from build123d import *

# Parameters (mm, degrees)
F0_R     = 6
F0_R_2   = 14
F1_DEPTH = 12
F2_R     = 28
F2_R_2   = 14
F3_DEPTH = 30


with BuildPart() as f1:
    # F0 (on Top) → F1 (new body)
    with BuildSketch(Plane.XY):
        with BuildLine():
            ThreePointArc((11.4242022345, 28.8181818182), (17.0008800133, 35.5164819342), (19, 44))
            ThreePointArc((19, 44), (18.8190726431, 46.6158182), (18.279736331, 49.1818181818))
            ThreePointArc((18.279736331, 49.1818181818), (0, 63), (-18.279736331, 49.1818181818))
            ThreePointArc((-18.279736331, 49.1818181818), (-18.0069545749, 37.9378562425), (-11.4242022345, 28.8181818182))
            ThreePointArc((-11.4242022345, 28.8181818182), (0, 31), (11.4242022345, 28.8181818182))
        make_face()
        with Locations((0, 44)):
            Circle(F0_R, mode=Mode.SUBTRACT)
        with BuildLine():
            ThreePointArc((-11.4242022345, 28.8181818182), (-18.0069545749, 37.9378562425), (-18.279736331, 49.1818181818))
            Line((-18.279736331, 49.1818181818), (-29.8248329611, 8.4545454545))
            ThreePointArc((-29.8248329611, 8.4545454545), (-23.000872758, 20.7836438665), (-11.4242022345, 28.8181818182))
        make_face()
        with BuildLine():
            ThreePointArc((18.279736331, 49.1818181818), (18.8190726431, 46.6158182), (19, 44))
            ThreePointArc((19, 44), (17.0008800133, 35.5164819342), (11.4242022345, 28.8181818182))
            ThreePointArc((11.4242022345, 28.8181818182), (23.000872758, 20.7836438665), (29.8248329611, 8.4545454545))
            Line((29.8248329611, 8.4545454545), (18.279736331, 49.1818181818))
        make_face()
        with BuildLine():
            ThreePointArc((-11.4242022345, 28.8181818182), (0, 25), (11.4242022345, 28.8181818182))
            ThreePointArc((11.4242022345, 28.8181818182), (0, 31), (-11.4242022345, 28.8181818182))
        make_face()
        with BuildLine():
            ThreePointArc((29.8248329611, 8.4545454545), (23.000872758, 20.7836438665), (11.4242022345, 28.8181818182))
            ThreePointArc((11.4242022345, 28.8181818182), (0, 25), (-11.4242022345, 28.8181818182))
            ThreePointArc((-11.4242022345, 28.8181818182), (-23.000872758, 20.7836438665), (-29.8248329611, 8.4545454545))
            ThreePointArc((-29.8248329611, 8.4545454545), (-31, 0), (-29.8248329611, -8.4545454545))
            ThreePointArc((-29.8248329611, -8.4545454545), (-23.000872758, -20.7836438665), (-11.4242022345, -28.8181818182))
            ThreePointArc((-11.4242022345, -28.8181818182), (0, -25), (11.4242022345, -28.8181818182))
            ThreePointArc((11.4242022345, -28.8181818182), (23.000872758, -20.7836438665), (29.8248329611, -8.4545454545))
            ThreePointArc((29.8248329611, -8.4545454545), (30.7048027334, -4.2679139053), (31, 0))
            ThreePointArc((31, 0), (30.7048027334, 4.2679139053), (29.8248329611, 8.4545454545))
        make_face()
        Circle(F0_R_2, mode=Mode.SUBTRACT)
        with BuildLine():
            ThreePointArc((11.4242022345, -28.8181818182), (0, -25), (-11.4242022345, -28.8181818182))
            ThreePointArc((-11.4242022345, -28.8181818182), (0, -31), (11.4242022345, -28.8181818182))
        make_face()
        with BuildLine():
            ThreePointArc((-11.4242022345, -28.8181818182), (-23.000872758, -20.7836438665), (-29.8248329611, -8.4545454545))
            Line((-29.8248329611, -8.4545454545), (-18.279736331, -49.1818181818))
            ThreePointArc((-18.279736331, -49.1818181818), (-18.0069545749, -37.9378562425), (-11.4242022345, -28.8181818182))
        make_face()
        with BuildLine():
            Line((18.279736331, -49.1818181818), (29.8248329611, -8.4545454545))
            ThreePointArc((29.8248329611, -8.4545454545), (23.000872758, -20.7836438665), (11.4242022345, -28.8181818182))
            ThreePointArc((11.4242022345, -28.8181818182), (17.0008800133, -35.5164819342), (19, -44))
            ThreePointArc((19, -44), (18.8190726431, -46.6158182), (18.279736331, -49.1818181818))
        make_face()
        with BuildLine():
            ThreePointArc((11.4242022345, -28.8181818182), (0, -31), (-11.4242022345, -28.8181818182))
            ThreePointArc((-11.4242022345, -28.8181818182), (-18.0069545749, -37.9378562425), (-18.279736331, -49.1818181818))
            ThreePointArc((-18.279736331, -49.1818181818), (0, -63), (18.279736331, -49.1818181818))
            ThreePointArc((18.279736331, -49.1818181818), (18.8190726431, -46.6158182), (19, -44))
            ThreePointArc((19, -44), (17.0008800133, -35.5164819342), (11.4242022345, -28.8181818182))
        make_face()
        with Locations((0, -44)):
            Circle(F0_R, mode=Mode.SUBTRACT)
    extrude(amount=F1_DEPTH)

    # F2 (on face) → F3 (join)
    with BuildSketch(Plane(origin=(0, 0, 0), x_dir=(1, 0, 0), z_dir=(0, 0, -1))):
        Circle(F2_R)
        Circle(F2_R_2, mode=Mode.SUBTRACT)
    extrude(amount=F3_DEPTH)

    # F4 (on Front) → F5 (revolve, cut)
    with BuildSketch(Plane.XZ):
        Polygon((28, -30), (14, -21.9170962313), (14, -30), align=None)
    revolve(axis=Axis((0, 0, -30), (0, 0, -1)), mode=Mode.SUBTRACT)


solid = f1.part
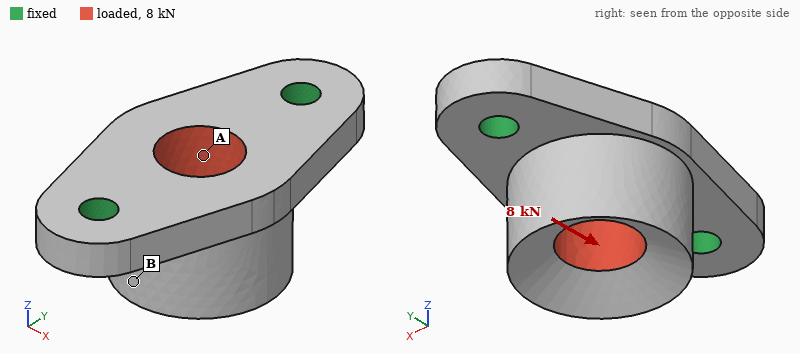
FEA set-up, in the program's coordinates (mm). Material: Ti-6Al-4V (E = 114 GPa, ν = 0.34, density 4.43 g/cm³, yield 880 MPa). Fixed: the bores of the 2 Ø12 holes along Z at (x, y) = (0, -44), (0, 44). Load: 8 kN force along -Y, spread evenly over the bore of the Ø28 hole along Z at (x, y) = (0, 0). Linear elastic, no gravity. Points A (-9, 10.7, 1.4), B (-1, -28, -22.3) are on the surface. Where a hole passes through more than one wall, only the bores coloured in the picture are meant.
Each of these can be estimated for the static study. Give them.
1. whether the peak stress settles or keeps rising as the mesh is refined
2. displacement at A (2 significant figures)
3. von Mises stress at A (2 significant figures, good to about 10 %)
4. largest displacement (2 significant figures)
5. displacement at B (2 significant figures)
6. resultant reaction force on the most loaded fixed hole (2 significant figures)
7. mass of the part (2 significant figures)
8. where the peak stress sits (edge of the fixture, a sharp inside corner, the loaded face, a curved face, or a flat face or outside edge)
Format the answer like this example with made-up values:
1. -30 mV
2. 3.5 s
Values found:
1. keeps rising
2. 2.6 µm
3. 6.4 MPa
4. 6.2 µm
5. 5.5 µm
6. 4.2 kN
7. 470 g
8. edge of the fixture
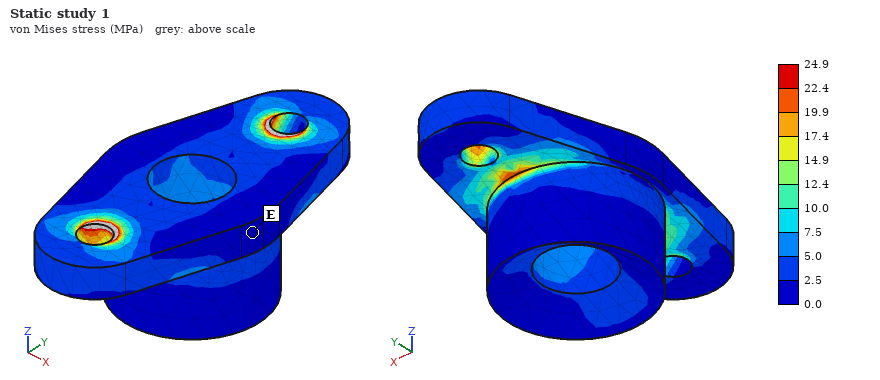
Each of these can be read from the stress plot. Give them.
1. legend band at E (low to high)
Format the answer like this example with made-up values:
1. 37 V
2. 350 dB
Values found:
1. 0.0 to 2.5 MPa
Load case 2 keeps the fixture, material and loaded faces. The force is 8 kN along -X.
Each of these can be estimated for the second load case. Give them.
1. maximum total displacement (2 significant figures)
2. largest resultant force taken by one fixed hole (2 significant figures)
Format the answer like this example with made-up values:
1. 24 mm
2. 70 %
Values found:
1. 41 µm
2. 4.0 kN
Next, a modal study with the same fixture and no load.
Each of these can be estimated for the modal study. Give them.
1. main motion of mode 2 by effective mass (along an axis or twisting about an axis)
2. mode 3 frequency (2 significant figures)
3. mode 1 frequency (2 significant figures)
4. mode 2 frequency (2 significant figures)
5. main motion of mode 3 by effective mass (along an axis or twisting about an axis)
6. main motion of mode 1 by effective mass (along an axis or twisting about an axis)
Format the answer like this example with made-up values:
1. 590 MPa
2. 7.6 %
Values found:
1. along Z
2. 10 kHz
3. 3700 Hz
4. 6800 Hz
5. along Y
6. along X
